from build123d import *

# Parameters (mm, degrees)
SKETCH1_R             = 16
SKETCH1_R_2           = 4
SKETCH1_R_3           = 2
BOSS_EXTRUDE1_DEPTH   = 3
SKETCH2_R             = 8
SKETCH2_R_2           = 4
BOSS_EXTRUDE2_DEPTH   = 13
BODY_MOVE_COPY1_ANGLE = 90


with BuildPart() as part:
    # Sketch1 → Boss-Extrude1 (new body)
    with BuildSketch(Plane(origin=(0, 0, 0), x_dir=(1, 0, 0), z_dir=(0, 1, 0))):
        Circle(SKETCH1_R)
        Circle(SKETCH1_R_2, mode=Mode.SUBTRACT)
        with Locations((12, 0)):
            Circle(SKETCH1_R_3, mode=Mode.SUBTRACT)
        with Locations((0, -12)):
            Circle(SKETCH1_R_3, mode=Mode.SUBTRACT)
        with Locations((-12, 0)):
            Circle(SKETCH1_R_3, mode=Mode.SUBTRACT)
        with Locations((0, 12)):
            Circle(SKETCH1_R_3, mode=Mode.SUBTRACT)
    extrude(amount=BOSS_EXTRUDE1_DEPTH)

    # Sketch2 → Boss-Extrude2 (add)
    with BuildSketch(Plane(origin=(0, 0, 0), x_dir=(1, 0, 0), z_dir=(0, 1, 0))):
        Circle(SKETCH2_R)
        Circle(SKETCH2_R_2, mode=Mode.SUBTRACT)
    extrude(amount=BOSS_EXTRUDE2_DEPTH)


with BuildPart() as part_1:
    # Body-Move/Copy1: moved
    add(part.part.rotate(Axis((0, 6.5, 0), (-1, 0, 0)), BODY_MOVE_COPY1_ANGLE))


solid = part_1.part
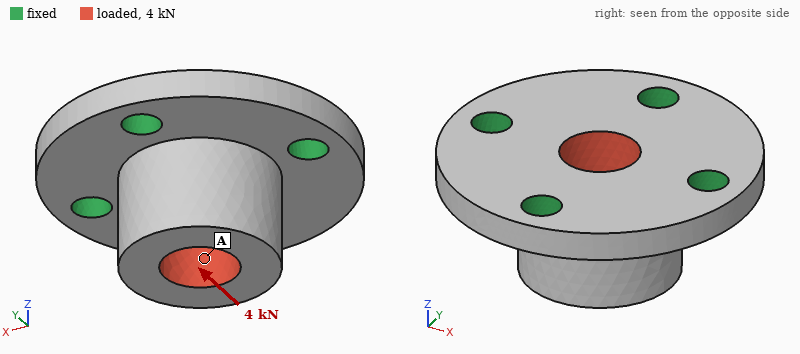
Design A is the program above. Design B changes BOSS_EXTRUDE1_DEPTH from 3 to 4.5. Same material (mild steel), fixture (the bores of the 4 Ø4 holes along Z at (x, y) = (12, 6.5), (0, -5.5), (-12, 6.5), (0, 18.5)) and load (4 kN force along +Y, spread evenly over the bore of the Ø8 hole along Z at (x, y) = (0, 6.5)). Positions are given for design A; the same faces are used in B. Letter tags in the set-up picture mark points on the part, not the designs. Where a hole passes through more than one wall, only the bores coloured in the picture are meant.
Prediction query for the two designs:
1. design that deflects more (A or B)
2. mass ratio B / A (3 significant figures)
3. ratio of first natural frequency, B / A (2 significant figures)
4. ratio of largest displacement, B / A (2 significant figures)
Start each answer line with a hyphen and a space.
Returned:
- A
- 1.23
- 1.4
- 0.56
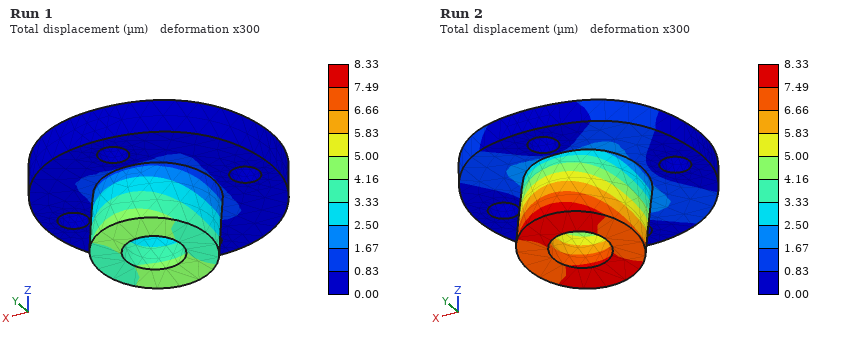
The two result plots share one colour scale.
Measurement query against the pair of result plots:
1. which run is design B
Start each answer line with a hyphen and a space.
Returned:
- Run 1
